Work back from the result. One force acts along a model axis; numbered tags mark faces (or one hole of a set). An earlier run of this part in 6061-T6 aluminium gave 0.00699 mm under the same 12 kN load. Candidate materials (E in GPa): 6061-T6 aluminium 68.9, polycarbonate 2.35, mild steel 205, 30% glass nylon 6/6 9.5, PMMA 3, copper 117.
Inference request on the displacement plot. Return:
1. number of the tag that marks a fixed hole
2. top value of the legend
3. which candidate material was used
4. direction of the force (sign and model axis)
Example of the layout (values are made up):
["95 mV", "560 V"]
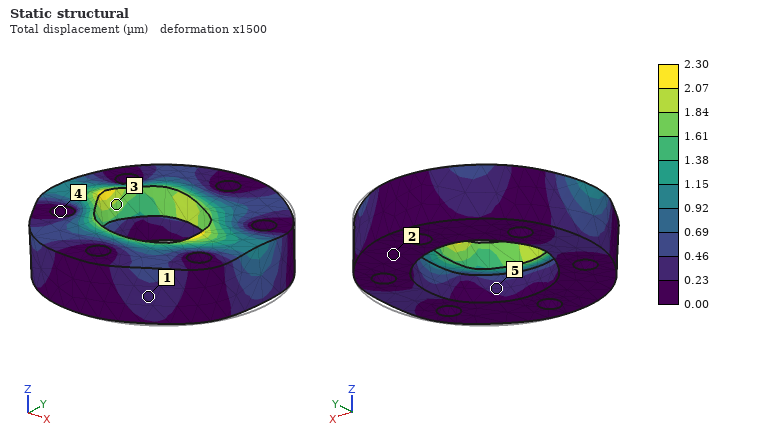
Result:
["4", "2.30 µm", "mild steel", "-X"]
